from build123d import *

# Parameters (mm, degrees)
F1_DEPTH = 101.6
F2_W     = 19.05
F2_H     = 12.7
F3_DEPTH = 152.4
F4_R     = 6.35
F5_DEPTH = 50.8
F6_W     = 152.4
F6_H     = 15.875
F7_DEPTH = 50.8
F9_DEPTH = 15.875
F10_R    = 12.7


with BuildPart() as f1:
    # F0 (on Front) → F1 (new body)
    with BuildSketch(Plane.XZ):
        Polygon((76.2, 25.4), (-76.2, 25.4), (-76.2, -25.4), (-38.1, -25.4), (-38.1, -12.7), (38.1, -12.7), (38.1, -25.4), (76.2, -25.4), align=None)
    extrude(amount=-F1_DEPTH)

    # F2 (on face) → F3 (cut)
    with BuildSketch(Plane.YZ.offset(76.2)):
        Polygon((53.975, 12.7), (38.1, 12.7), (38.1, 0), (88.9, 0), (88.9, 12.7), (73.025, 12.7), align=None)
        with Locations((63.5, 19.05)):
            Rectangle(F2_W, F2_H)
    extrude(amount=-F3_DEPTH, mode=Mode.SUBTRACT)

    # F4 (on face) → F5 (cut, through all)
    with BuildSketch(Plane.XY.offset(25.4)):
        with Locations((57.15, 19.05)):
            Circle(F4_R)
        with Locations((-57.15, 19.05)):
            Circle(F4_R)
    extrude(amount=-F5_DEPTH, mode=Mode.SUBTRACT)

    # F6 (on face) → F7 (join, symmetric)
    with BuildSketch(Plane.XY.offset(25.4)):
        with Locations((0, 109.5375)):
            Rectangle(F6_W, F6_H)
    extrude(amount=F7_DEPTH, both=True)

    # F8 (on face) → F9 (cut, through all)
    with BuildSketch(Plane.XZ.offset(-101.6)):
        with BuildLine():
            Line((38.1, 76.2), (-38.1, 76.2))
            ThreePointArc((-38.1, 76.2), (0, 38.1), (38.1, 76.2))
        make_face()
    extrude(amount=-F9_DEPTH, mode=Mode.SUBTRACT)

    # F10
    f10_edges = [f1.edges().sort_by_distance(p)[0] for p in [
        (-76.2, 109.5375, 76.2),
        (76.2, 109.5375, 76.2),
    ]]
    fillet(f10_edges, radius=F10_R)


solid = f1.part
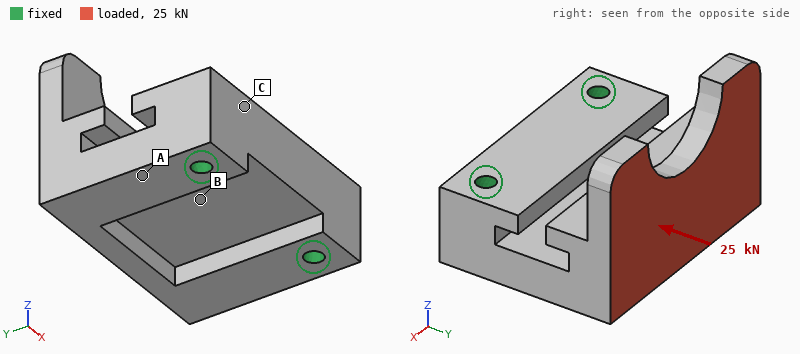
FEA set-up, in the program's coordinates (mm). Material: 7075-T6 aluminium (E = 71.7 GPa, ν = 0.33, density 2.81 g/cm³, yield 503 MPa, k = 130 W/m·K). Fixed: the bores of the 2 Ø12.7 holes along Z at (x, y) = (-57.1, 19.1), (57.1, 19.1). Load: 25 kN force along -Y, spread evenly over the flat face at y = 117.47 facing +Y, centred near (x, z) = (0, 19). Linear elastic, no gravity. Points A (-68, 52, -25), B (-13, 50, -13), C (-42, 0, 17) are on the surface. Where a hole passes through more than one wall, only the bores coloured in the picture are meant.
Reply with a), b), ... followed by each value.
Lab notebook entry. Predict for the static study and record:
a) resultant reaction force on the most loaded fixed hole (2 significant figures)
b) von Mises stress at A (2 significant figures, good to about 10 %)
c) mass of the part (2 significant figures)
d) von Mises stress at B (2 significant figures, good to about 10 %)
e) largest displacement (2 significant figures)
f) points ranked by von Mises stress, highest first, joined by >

a) 13 kN
b) 65 MPa
c) 2.1 kg
d) 28 MPa
e) 0.69 mm
f) A > B > C
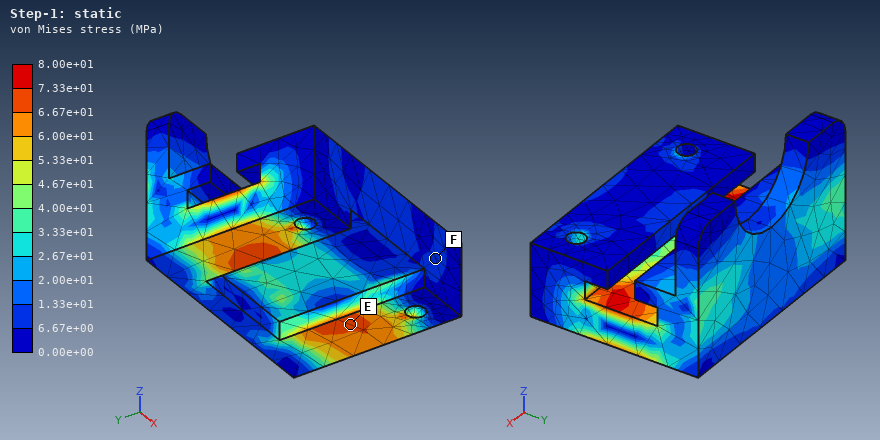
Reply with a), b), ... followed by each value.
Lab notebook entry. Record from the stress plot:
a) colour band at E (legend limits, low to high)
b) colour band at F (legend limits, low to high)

a) 6.67e+01 to 7.33e+01 MPa
b) 6.67e+00 to 1.33e+01 MPa
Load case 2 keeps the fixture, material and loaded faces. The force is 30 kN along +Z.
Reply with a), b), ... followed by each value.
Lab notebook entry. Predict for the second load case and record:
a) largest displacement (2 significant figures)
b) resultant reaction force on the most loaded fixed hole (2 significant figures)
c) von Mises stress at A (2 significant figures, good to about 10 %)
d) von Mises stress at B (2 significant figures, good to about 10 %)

a) 1.4 mm
b) 16 kN
c) 190 MPa
d) 95 MPa
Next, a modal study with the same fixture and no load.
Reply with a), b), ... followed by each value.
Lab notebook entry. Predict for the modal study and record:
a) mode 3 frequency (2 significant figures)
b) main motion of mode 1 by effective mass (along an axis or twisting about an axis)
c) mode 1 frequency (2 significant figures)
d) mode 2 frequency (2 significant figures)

a) 3000 Hz
b) along Z
c) 1000 Hz
d) 1800 Hz
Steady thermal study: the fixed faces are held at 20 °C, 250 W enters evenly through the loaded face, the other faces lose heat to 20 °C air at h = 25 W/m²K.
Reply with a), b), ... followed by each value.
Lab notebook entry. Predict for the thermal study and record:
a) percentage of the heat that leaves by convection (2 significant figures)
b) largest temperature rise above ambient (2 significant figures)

a) 20 %
b) 60 K
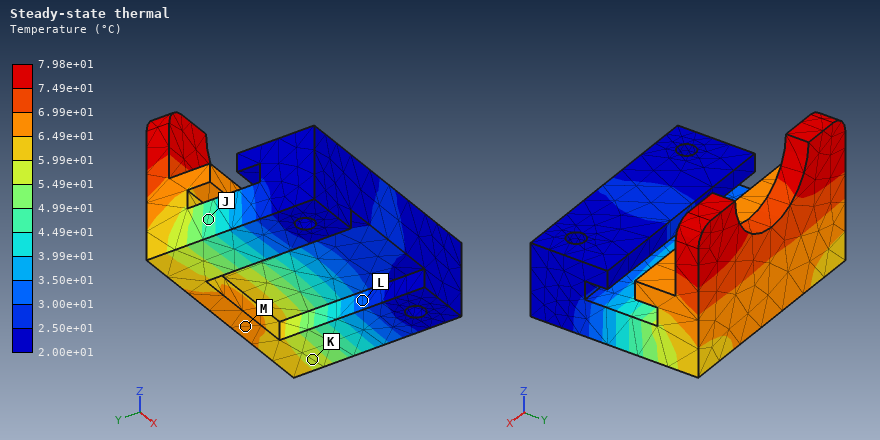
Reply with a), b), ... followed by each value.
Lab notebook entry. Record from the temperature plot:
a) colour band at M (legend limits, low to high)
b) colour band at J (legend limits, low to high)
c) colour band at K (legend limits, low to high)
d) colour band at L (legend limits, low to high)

a) 6.49e+01 to 6.99e+01 °C
b) 4.49e+01 to 4.99e+01 °C
c) 5.49e+01 to 5.99e+01 °C
d) 3.00e+01 to 3.50e+01 °C
